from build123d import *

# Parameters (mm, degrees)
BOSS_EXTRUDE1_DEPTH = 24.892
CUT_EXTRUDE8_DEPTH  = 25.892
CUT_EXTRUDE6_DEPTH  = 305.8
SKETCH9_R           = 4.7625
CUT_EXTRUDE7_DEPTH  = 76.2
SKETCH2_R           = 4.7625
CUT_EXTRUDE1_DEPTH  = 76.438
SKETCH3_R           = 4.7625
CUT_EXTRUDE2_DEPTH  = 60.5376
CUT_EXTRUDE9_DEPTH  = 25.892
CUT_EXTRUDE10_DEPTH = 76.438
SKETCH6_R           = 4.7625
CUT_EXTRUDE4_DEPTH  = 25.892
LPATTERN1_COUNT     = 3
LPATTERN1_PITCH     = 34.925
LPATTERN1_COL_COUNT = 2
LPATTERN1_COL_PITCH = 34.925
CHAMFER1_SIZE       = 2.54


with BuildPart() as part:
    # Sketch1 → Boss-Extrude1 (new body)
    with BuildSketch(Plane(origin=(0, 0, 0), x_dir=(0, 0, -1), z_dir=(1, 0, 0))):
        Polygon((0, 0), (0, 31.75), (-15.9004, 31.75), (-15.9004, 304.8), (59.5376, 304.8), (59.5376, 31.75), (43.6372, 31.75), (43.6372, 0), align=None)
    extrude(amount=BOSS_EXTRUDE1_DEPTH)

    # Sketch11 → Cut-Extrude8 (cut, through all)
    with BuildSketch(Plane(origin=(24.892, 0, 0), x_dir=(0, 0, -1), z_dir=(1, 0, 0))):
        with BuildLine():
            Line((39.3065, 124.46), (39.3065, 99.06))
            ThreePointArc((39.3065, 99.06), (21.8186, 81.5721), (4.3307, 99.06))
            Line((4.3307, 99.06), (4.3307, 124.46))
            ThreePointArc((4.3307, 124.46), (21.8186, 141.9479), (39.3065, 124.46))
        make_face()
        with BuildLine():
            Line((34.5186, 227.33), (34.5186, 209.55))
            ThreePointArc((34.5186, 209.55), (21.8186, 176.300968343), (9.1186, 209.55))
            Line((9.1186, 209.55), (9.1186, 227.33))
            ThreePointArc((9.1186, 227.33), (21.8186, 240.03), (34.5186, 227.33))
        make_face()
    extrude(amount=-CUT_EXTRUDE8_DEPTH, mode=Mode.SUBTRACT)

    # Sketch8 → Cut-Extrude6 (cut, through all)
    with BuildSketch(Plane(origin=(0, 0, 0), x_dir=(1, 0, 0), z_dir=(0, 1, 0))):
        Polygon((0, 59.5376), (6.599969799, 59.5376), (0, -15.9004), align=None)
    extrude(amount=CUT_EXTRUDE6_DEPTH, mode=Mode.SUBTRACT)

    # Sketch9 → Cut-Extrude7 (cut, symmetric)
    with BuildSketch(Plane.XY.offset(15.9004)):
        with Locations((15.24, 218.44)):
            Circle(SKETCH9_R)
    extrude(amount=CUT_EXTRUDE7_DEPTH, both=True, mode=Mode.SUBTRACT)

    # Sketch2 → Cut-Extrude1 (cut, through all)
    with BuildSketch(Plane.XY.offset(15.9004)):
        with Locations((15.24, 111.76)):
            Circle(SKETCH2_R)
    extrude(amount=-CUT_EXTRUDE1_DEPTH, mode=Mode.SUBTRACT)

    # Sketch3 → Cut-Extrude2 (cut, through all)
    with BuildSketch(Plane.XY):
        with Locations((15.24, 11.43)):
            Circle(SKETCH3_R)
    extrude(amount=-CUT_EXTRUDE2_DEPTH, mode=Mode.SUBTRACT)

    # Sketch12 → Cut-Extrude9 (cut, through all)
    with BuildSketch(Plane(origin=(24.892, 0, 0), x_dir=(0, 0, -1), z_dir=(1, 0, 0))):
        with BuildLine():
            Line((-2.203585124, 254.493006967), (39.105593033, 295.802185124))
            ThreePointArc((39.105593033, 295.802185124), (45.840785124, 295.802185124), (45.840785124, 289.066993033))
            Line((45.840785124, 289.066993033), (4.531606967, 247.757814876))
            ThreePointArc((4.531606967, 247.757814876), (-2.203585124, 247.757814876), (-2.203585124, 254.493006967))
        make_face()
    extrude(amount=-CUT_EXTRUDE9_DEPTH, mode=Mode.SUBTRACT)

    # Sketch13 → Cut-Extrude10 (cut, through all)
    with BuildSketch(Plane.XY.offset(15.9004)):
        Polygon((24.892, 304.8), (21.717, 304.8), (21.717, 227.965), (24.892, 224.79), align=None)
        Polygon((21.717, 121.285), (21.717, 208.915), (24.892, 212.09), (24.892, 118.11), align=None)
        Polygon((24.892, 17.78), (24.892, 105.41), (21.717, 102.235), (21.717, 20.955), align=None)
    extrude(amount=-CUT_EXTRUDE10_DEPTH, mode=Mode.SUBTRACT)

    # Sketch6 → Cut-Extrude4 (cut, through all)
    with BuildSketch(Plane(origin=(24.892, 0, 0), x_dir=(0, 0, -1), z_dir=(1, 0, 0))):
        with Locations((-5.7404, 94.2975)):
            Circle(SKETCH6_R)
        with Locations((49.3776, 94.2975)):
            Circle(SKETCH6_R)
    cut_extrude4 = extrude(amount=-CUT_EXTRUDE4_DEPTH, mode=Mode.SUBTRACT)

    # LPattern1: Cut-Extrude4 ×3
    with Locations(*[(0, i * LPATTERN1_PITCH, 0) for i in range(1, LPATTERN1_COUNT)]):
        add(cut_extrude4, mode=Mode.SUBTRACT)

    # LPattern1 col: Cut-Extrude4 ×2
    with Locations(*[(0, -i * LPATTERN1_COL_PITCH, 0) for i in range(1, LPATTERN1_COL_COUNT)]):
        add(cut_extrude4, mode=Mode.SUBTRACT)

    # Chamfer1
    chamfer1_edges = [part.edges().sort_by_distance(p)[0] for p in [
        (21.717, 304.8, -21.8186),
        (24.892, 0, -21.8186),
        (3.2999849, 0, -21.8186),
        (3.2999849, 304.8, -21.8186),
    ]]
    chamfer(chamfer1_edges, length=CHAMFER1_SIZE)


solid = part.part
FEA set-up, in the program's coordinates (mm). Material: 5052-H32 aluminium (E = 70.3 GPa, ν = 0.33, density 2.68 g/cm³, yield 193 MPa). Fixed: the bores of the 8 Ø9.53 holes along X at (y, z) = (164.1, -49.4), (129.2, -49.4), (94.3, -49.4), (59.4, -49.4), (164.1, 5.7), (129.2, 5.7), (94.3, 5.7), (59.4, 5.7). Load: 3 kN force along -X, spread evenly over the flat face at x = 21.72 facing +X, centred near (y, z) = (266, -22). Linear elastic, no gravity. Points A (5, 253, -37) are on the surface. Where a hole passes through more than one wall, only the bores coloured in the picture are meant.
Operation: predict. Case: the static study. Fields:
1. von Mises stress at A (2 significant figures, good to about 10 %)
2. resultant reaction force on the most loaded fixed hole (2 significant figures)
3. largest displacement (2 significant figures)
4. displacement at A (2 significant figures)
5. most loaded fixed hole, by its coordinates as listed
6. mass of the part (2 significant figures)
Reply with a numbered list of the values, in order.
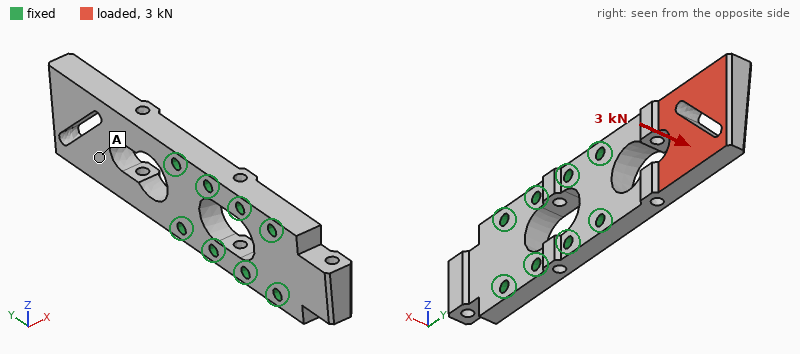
1. 13 MPa
2. 2.7 kN
3. 1.00 mm
4. 0.51 mm
5. (164.1, 5.7)
6. 840 g
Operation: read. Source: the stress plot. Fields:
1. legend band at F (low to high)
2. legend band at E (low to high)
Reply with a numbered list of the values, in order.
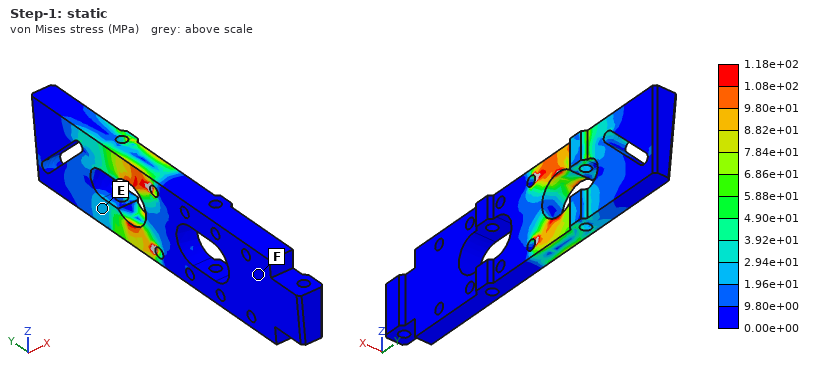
1. 0.00e+00 to 9.80e+00 MPa
2. 1.96e+01 to 2.94e+01 MPa
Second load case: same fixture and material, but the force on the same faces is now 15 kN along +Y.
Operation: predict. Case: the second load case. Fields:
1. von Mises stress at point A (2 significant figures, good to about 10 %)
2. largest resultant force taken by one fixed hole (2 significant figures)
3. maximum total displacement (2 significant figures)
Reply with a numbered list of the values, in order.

1. 15 MPa
2. 7.1 kN
3. 0.70 mm
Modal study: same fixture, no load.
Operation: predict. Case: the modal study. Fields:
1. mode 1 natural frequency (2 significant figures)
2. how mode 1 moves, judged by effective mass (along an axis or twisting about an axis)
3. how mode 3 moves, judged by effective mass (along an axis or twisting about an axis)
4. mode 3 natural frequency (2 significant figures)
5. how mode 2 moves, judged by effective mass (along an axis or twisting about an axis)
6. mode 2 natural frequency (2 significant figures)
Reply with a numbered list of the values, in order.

1. 660 Hz
2. along X
3. twisting about Y
4. 2100 Hz
5. along Z
6. 1900 Hz
